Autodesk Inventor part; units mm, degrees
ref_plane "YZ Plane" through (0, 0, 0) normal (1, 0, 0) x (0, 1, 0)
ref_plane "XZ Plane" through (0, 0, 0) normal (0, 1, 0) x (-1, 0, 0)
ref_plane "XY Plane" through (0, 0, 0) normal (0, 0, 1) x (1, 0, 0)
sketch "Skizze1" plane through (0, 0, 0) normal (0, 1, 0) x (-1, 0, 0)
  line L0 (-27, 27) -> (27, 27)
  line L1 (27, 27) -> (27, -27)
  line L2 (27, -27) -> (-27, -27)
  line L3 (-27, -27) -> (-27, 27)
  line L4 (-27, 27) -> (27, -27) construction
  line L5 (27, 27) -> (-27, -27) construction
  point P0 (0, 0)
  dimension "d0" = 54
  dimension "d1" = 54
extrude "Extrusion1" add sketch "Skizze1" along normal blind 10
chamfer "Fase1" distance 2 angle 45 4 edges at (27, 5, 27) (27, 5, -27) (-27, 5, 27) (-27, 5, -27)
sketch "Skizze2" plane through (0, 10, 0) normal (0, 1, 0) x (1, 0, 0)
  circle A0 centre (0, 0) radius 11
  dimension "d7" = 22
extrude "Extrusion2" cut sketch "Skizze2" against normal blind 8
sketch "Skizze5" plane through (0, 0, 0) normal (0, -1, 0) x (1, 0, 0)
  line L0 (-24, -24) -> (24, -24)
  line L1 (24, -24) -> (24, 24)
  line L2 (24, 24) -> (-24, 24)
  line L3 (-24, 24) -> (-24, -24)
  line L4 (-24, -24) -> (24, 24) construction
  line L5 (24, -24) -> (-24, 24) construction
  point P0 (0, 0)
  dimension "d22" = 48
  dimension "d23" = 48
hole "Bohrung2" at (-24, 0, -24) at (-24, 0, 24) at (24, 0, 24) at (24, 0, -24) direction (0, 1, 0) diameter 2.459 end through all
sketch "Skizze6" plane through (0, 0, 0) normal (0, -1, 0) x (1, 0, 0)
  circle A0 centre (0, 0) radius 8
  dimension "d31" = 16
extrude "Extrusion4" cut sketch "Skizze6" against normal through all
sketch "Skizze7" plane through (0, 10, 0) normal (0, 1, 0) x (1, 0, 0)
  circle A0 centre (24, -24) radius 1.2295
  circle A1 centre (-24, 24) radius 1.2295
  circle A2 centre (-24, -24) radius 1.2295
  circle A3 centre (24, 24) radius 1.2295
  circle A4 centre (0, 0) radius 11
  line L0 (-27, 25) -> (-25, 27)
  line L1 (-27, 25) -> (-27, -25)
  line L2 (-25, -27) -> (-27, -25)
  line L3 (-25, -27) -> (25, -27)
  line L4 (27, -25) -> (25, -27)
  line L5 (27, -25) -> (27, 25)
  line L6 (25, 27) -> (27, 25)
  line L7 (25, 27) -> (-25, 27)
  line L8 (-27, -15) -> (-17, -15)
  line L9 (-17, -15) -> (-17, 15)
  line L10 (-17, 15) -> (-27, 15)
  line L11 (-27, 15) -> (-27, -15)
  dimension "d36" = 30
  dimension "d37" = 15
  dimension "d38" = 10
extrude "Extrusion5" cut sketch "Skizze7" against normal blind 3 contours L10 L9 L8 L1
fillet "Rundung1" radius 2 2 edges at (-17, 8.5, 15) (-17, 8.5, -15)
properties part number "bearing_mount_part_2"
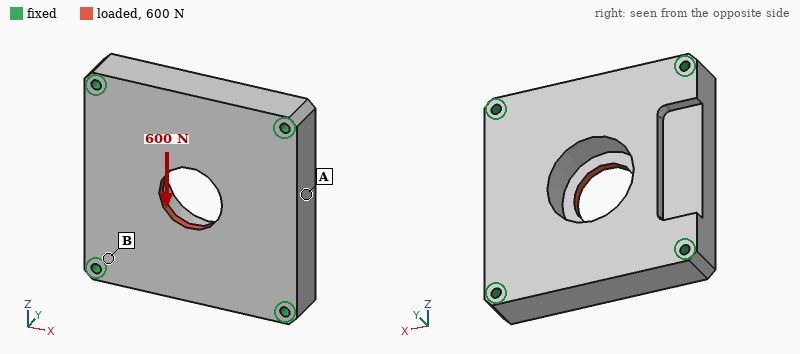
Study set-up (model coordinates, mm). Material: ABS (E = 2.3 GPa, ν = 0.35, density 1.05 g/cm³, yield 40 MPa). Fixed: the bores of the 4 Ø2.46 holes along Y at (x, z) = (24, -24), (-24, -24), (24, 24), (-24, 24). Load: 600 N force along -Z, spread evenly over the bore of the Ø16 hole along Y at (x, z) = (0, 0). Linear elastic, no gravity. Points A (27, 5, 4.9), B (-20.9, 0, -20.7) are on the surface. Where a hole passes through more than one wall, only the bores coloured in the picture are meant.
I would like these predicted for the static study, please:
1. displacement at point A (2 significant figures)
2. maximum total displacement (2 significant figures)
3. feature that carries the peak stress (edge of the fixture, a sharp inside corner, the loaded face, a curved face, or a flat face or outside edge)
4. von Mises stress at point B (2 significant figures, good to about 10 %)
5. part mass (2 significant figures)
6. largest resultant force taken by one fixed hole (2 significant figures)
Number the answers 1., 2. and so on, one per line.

1. 8.6 µm
2. 50 µm
3. a sharp inside corner
4. 2.4 MPa
5. 26 g
6. 180 N
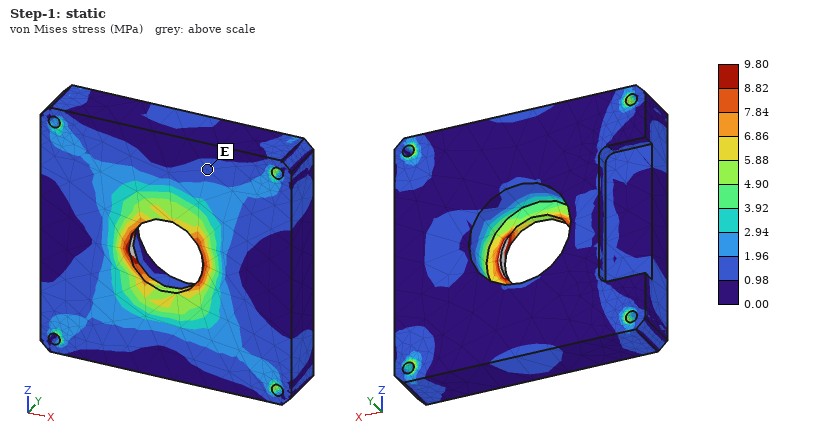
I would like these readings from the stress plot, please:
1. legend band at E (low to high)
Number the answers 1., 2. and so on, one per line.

1. 0.98 to 1.96 MPa
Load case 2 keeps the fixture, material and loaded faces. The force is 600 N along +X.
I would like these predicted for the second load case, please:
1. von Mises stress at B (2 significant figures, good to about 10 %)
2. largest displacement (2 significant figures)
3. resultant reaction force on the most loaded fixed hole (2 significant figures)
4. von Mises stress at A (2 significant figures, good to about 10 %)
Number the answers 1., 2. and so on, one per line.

1. 2.1 MPa
2. 49 µm
3. 170 N
4. 0.99 MPa
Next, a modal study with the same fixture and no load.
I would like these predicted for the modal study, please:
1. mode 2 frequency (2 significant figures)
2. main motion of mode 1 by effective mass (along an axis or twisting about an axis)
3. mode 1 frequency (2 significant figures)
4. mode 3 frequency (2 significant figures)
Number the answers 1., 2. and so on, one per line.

1. 4900 Hz
2. along Y
3. 3300 Hz
4. 5000 Hz
